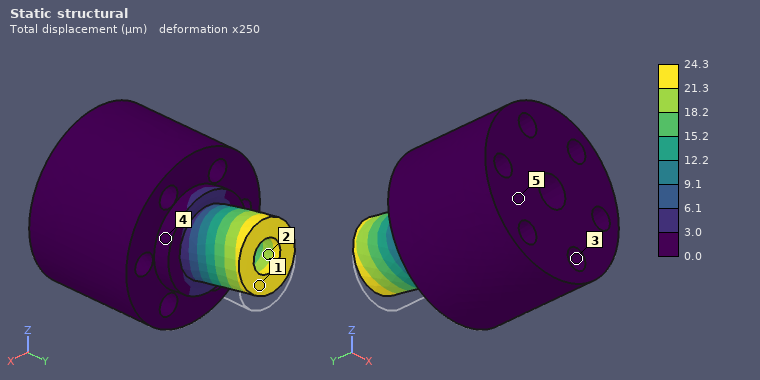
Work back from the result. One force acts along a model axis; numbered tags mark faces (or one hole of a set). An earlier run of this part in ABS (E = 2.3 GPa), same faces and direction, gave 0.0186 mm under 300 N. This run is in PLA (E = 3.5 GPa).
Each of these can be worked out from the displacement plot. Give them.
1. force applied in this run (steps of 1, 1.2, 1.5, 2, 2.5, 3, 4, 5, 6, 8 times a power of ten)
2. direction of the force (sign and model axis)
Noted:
600 N
+Z
